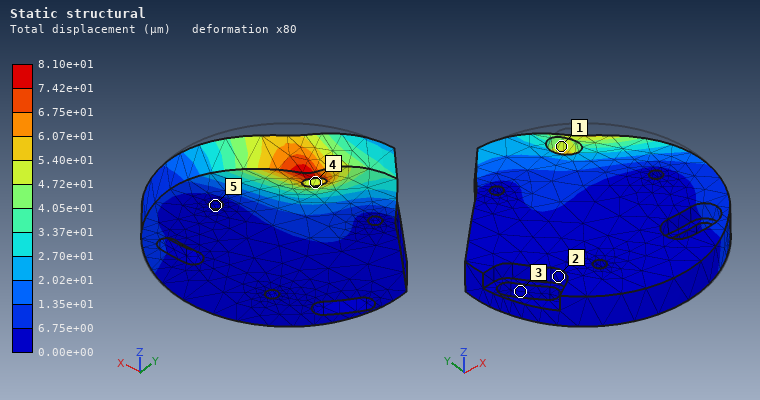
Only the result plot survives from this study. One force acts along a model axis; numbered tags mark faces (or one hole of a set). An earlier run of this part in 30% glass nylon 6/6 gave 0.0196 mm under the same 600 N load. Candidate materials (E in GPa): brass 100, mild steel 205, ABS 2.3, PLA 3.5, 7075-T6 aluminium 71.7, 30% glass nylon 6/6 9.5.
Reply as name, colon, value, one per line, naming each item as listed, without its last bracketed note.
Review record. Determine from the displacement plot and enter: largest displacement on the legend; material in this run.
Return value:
largest displacement on the legend: 8.10e+01 µm
material in this run: ABS
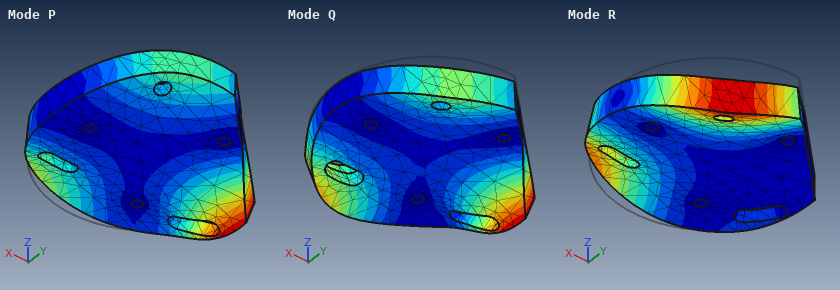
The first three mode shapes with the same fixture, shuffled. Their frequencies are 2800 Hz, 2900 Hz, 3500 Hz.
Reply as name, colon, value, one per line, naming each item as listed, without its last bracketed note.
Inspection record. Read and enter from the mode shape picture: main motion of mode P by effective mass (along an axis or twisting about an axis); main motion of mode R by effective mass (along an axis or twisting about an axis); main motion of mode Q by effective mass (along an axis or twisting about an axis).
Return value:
main motion of mode P by effective mass: twisting about Y
main motion of mode R by effective mass: twisting about X
main motion of mode Q by effective mass: along Z
